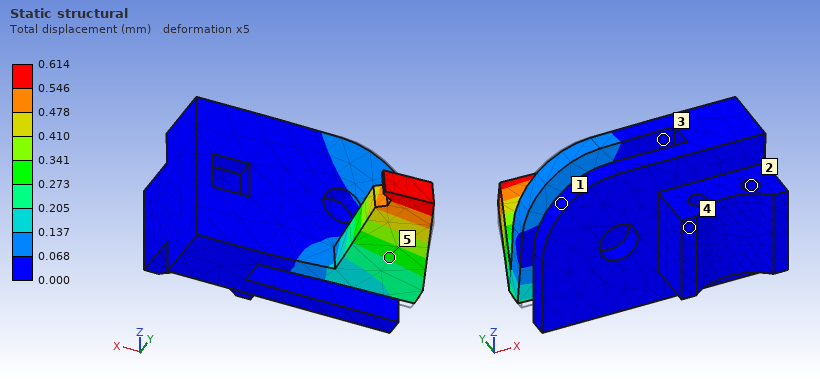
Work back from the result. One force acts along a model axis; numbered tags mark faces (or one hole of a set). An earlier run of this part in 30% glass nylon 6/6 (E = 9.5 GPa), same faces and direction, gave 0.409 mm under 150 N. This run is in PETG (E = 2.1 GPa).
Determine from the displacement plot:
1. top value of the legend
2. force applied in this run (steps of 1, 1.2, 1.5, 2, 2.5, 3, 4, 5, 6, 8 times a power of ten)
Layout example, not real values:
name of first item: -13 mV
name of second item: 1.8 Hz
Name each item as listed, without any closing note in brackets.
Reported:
top value of the legend: 0.614 mm
force applied in this run: 50 N
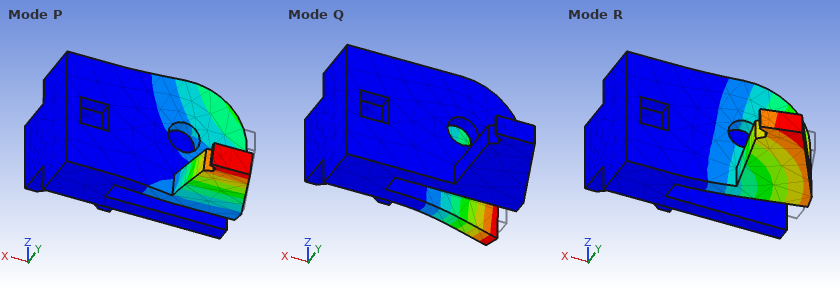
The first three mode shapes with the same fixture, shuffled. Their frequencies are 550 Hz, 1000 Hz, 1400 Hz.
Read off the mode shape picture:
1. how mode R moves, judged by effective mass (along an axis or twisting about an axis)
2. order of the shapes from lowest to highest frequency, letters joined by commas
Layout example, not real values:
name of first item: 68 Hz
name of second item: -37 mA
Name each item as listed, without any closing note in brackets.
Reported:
how mode R moves, judged by effective mass: along Y
order of the shapes from lowest to highest frequency, letters joined by commas: R, P, Q
